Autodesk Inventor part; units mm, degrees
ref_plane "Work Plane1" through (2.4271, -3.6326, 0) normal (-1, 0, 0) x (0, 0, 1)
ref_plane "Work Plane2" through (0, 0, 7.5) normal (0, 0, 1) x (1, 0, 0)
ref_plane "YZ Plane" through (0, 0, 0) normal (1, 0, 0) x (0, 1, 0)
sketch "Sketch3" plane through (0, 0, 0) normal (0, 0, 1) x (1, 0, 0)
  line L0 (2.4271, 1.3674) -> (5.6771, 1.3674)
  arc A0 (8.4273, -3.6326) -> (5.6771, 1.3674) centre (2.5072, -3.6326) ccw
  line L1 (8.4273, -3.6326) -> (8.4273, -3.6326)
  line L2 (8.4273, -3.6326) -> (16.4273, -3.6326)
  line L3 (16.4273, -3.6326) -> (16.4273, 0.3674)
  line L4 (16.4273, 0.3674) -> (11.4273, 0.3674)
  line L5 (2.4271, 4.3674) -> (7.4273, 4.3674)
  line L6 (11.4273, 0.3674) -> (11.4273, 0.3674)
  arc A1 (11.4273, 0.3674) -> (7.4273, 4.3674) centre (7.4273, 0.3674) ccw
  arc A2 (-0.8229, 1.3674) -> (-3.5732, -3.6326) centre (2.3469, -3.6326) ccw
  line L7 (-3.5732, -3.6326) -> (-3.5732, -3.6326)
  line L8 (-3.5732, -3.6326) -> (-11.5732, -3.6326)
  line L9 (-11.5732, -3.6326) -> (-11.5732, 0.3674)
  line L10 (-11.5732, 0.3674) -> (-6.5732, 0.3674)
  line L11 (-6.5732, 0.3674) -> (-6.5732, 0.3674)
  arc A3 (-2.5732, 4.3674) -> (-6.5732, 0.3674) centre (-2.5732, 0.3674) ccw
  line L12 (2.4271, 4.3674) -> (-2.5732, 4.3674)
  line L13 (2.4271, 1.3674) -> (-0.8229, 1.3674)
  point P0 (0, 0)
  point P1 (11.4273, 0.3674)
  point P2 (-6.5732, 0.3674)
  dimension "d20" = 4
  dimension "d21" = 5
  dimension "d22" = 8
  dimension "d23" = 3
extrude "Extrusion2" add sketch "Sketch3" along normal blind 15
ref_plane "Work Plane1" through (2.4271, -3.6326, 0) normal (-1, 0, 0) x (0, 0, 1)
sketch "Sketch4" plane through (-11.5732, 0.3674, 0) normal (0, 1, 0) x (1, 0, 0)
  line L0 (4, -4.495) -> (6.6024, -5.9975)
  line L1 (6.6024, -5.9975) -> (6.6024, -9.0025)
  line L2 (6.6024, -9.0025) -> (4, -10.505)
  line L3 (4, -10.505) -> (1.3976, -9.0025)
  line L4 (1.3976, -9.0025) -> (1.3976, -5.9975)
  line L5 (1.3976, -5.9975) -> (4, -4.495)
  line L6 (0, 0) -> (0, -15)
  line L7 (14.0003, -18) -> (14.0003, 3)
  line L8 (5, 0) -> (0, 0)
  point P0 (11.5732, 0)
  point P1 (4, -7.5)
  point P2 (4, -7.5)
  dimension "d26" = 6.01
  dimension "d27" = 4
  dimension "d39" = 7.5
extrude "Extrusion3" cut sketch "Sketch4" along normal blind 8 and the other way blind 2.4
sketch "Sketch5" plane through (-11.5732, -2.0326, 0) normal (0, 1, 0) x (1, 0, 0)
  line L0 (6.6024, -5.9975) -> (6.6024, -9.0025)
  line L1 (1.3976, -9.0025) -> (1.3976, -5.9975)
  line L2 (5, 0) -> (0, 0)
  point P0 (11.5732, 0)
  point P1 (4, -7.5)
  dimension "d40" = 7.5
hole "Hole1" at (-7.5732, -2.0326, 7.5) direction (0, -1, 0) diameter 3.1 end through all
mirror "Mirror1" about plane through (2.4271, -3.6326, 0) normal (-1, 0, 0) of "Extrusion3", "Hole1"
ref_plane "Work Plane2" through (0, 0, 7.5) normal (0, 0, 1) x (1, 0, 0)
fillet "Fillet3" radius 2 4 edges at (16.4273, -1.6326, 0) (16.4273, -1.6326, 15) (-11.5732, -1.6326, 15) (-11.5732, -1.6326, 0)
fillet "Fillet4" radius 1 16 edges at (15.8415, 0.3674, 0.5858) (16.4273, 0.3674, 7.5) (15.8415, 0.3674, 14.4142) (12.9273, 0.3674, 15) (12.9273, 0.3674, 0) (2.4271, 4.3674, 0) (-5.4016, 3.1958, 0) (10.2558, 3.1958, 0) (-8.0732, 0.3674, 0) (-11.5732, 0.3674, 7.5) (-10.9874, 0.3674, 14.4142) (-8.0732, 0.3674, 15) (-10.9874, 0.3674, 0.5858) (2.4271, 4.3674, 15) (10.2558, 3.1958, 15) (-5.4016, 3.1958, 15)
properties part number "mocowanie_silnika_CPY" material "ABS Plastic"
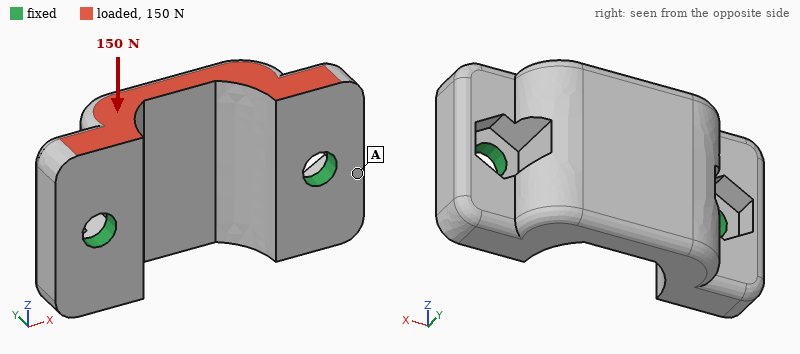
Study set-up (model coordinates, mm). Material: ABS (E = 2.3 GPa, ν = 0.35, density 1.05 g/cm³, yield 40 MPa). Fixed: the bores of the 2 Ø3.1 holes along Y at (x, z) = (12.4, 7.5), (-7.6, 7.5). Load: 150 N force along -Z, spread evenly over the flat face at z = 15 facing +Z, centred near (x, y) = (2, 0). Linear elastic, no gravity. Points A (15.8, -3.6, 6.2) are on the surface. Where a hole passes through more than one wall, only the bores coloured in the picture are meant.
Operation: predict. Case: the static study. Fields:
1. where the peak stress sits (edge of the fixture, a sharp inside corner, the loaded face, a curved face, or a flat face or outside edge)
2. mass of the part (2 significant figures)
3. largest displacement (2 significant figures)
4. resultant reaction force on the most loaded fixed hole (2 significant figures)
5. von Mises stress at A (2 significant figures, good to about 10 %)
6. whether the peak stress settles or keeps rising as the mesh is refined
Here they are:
edge of the fixture
1.8 g
0.15 mm
75 N
4.9 MPa
keeps rising
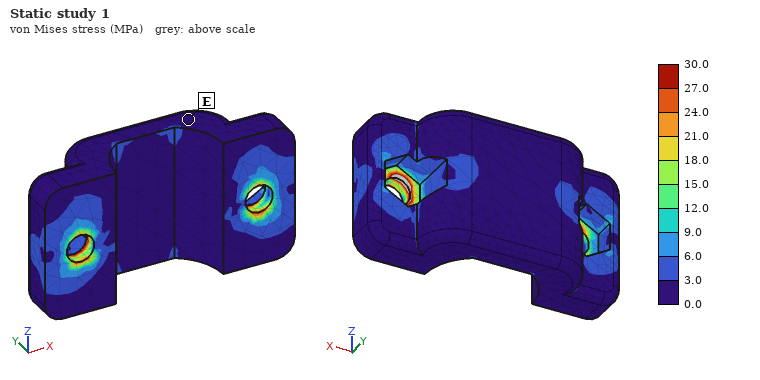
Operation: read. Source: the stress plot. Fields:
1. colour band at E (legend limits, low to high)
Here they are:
0.0 to 3.0 MPa
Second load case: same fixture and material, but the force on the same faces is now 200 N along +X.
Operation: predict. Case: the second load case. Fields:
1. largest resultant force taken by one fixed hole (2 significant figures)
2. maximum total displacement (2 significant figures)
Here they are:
110 N
0.10 mm
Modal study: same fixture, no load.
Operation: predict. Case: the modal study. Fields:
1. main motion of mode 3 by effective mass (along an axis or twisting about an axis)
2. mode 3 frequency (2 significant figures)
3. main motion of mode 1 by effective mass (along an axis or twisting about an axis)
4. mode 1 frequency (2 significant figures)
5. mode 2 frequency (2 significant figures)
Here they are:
along X
10 kHz
along Z
3700 Hz
8400 Hz
